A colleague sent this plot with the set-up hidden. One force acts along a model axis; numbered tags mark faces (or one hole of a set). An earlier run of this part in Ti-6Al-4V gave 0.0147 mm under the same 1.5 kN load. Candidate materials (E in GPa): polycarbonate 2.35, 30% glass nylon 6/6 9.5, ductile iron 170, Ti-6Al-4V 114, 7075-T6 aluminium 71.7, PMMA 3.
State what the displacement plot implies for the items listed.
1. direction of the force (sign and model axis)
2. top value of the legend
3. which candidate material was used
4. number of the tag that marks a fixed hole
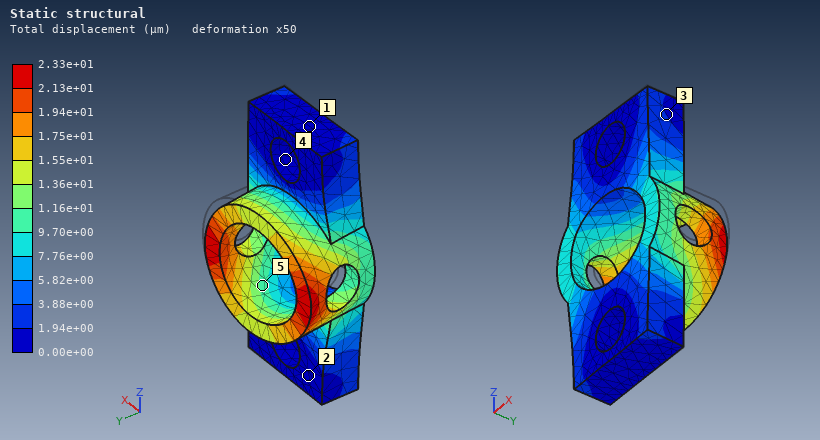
-X
2.33e+01 µm
7075-T6 aluminium
4
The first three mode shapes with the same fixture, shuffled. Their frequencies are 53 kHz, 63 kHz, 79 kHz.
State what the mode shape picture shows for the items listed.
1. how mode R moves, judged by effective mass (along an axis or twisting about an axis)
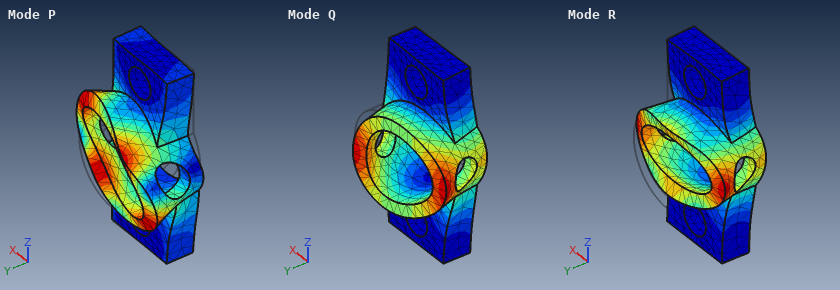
along Y
